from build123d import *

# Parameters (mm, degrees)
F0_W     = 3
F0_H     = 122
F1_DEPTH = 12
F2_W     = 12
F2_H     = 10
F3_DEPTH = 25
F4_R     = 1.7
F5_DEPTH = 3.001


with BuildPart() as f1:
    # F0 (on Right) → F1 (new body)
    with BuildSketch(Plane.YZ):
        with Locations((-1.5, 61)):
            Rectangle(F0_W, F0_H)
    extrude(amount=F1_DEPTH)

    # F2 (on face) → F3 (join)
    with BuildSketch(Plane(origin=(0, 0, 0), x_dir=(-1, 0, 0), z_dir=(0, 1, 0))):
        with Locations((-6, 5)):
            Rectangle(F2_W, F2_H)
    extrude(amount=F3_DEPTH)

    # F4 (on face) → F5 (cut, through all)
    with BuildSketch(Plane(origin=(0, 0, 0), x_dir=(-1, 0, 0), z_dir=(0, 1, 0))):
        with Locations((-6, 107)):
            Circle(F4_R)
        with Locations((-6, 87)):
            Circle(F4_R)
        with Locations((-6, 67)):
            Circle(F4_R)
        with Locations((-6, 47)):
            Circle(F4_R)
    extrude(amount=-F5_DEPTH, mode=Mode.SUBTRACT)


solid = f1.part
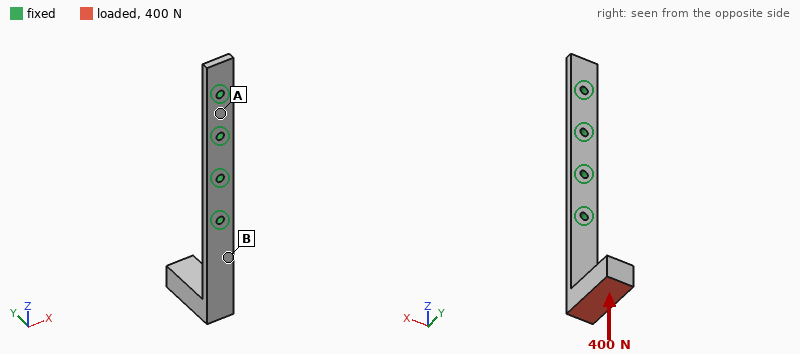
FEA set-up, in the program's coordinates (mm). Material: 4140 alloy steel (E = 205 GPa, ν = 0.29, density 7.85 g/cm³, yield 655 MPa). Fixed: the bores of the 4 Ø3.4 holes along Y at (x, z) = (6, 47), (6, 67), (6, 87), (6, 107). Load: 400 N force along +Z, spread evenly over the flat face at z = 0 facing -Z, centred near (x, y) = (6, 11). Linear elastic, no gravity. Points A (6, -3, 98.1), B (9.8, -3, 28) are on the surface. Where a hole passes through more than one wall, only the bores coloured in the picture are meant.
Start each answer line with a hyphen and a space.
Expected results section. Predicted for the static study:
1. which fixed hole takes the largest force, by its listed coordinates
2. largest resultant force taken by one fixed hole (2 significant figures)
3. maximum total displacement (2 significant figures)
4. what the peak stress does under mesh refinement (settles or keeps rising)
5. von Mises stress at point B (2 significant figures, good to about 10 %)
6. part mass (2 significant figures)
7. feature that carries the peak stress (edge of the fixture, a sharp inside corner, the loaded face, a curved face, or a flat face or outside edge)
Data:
- (6, 47)
- 370 N
- 1.3 mm
- keeps rising
- 270 MPa
- 57 g
- edge of the fixture
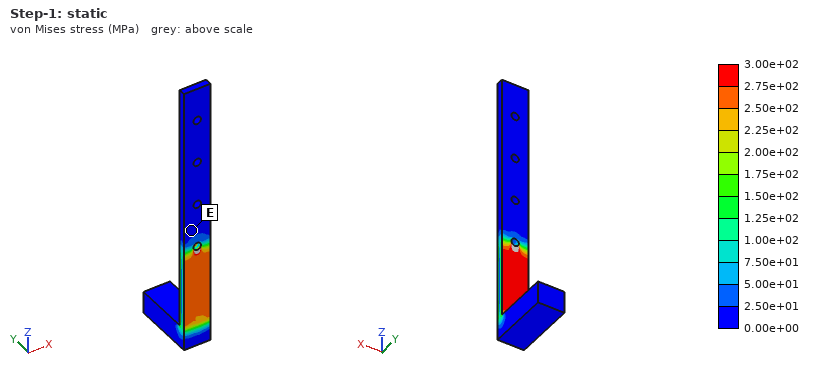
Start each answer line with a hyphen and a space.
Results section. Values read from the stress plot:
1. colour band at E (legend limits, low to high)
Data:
- 0.00e+00 to 2.50e+01 MPa
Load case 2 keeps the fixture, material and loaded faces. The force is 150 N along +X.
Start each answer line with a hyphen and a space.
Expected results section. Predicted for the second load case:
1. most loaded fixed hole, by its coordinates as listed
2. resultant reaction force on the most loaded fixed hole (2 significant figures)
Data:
- (6, 47)
- 350 N
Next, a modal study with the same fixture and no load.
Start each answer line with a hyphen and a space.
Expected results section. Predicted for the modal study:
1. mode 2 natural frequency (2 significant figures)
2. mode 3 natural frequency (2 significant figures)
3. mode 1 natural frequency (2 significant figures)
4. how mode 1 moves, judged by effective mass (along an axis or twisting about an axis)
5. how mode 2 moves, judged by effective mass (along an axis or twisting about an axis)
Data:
- 820 Hz
- 1900 Hz
- 410 Hz
- along Y
- along X
